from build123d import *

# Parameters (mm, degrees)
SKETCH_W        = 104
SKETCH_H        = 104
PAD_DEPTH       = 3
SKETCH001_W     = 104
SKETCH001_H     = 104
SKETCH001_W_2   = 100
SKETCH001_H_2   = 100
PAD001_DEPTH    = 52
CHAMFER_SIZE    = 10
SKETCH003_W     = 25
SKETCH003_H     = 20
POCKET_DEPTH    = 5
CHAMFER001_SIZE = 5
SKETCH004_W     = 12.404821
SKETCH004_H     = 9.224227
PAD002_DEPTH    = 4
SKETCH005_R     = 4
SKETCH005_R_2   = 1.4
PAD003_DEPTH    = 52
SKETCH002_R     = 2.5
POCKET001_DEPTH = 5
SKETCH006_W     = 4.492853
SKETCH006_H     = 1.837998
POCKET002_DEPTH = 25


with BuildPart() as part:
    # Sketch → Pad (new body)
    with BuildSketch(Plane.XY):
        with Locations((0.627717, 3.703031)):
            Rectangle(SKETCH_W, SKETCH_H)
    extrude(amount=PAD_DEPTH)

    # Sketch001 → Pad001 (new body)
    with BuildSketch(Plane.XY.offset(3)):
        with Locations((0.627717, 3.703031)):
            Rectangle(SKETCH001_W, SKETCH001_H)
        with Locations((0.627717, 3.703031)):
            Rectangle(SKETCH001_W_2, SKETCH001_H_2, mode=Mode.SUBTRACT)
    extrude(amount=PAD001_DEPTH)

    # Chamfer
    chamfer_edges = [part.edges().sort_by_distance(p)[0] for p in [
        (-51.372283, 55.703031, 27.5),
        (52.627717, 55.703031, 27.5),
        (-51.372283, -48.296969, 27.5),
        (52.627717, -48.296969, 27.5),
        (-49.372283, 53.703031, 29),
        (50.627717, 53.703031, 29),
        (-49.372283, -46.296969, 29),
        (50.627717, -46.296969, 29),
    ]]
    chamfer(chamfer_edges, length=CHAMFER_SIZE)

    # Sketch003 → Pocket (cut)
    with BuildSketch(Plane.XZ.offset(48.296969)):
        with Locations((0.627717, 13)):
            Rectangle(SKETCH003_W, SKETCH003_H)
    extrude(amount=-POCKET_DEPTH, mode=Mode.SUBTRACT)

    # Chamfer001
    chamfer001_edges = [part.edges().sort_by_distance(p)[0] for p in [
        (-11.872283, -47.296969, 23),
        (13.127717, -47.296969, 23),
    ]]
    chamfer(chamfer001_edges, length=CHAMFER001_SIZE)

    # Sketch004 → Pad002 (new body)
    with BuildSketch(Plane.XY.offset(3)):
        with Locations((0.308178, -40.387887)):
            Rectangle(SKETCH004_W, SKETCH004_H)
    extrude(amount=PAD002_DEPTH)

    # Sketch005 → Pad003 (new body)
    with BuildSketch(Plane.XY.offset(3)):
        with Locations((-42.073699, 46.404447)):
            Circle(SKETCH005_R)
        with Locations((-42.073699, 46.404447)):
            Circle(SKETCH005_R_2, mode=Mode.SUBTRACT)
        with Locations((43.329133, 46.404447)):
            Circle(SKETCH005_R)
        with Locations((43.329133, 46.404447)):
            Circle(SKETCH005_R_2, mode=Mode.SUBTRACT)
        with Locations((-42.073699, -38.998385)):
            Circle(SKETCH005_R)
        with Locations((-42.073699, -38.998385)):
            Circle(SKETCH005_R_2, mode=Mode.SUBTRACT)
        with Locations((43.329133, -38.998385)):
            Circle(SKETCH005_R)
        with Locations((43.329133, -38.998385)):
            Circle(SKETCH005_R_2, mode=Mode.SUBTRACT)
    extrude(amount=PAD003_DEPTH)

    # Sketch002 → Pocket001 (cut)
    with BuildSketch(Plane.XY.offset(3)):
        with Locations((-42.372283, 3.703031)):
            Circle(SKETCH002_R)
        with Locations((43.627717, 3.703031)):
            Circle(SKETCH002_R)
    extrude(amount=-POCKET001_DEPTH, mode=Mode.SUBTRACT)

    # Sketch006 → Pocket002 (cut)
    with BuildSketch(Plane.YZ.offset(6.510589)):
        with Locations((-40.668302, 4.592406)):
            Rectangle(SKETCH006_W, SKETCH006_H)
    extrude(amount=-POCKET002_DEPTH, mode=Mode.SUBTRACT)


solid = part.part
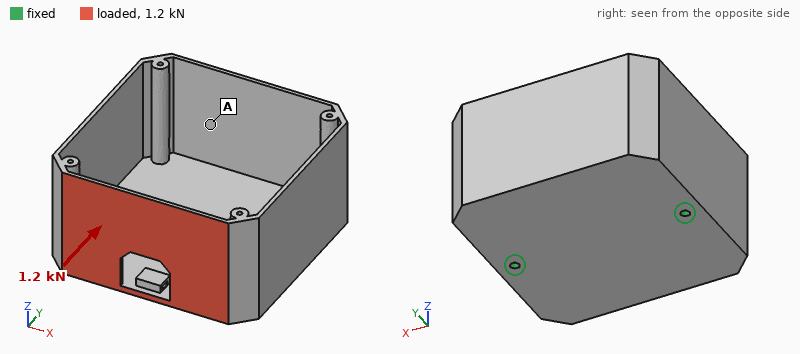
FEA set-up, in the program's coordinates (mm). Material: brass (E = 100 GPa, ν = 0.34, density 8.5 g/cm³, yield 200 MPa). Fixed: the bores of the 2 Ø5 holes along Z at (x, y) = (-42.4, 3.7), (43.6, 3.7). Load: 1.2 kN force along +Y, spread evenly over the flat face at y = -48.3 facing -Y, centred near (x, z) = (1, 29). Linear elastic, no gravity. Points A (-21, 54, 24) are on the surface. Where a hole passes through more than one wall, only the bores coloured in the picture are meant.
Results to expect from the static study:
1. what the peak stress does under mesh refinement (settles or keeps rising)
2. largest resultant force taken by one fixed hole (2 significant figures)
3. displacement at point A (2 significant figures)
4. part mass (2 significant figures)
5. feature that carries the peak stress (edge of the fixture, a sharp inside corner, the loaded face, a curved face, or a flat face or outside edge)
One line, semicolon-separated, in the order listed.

keeps rising; 610 N; 0.40 mm; 700 g; edge of the fixture
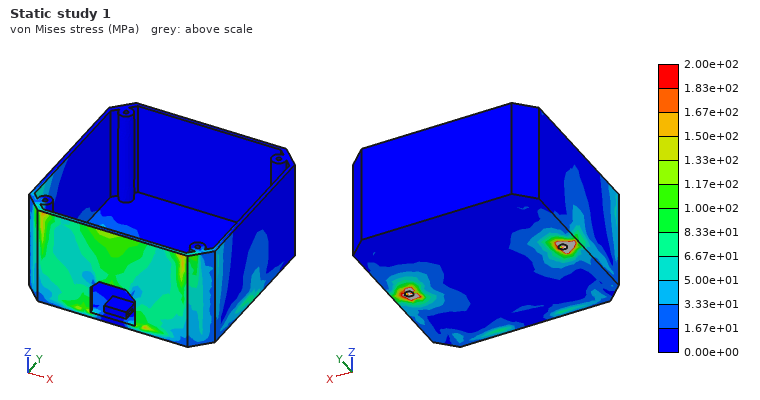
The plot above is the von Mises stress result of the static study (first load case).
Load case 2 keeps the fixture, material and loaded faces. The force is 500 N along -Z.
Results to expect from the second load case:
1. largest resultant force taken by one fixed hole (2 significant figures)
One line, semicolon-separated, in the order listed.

260 N
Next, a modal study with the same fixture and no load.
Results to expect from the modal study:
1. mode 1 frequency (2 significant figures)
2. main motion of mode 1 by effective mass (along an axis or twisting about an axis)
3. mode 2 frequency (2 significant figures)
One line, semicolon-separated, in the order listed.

290 Hz; along Y; 400 Hz
